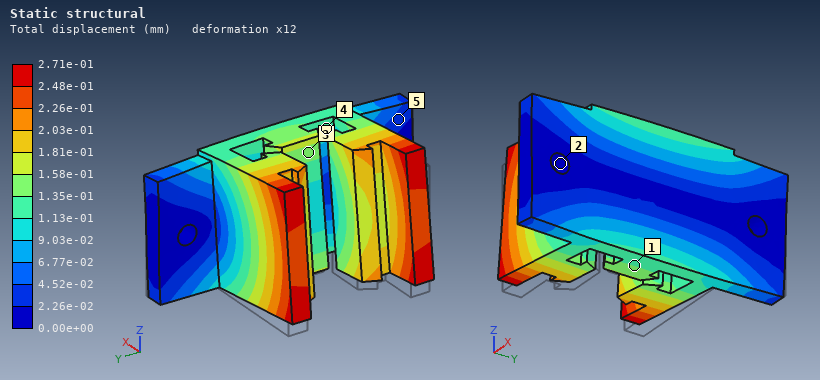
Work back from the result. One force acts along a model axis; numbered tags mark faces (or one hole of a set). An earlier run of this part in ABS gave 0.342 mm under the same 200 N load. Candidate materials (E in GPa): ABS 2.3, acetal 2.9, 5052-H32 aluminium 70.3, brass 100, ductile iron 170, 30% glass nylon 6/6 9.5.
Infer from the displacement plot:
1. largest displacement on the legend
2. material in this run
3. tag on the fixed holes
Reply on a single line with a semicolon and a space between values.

2.71e-01 mm; acetal; 2
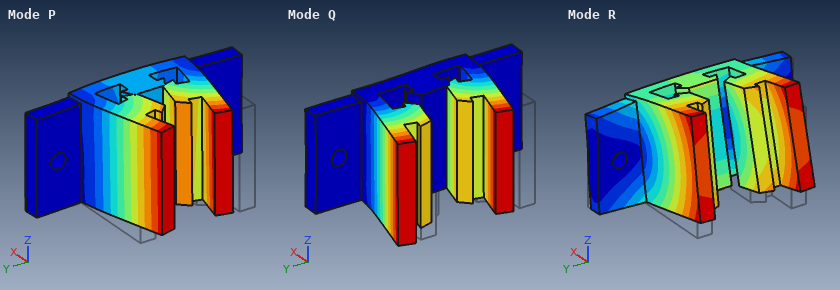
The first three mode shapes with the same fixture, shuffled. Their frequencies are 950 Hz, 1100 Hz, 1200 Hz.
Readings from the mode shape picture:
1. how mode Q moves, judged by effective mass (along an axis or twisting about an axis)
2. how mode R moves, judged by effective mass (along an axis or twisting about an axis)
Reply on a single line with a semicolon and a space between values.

along Y; along Z
